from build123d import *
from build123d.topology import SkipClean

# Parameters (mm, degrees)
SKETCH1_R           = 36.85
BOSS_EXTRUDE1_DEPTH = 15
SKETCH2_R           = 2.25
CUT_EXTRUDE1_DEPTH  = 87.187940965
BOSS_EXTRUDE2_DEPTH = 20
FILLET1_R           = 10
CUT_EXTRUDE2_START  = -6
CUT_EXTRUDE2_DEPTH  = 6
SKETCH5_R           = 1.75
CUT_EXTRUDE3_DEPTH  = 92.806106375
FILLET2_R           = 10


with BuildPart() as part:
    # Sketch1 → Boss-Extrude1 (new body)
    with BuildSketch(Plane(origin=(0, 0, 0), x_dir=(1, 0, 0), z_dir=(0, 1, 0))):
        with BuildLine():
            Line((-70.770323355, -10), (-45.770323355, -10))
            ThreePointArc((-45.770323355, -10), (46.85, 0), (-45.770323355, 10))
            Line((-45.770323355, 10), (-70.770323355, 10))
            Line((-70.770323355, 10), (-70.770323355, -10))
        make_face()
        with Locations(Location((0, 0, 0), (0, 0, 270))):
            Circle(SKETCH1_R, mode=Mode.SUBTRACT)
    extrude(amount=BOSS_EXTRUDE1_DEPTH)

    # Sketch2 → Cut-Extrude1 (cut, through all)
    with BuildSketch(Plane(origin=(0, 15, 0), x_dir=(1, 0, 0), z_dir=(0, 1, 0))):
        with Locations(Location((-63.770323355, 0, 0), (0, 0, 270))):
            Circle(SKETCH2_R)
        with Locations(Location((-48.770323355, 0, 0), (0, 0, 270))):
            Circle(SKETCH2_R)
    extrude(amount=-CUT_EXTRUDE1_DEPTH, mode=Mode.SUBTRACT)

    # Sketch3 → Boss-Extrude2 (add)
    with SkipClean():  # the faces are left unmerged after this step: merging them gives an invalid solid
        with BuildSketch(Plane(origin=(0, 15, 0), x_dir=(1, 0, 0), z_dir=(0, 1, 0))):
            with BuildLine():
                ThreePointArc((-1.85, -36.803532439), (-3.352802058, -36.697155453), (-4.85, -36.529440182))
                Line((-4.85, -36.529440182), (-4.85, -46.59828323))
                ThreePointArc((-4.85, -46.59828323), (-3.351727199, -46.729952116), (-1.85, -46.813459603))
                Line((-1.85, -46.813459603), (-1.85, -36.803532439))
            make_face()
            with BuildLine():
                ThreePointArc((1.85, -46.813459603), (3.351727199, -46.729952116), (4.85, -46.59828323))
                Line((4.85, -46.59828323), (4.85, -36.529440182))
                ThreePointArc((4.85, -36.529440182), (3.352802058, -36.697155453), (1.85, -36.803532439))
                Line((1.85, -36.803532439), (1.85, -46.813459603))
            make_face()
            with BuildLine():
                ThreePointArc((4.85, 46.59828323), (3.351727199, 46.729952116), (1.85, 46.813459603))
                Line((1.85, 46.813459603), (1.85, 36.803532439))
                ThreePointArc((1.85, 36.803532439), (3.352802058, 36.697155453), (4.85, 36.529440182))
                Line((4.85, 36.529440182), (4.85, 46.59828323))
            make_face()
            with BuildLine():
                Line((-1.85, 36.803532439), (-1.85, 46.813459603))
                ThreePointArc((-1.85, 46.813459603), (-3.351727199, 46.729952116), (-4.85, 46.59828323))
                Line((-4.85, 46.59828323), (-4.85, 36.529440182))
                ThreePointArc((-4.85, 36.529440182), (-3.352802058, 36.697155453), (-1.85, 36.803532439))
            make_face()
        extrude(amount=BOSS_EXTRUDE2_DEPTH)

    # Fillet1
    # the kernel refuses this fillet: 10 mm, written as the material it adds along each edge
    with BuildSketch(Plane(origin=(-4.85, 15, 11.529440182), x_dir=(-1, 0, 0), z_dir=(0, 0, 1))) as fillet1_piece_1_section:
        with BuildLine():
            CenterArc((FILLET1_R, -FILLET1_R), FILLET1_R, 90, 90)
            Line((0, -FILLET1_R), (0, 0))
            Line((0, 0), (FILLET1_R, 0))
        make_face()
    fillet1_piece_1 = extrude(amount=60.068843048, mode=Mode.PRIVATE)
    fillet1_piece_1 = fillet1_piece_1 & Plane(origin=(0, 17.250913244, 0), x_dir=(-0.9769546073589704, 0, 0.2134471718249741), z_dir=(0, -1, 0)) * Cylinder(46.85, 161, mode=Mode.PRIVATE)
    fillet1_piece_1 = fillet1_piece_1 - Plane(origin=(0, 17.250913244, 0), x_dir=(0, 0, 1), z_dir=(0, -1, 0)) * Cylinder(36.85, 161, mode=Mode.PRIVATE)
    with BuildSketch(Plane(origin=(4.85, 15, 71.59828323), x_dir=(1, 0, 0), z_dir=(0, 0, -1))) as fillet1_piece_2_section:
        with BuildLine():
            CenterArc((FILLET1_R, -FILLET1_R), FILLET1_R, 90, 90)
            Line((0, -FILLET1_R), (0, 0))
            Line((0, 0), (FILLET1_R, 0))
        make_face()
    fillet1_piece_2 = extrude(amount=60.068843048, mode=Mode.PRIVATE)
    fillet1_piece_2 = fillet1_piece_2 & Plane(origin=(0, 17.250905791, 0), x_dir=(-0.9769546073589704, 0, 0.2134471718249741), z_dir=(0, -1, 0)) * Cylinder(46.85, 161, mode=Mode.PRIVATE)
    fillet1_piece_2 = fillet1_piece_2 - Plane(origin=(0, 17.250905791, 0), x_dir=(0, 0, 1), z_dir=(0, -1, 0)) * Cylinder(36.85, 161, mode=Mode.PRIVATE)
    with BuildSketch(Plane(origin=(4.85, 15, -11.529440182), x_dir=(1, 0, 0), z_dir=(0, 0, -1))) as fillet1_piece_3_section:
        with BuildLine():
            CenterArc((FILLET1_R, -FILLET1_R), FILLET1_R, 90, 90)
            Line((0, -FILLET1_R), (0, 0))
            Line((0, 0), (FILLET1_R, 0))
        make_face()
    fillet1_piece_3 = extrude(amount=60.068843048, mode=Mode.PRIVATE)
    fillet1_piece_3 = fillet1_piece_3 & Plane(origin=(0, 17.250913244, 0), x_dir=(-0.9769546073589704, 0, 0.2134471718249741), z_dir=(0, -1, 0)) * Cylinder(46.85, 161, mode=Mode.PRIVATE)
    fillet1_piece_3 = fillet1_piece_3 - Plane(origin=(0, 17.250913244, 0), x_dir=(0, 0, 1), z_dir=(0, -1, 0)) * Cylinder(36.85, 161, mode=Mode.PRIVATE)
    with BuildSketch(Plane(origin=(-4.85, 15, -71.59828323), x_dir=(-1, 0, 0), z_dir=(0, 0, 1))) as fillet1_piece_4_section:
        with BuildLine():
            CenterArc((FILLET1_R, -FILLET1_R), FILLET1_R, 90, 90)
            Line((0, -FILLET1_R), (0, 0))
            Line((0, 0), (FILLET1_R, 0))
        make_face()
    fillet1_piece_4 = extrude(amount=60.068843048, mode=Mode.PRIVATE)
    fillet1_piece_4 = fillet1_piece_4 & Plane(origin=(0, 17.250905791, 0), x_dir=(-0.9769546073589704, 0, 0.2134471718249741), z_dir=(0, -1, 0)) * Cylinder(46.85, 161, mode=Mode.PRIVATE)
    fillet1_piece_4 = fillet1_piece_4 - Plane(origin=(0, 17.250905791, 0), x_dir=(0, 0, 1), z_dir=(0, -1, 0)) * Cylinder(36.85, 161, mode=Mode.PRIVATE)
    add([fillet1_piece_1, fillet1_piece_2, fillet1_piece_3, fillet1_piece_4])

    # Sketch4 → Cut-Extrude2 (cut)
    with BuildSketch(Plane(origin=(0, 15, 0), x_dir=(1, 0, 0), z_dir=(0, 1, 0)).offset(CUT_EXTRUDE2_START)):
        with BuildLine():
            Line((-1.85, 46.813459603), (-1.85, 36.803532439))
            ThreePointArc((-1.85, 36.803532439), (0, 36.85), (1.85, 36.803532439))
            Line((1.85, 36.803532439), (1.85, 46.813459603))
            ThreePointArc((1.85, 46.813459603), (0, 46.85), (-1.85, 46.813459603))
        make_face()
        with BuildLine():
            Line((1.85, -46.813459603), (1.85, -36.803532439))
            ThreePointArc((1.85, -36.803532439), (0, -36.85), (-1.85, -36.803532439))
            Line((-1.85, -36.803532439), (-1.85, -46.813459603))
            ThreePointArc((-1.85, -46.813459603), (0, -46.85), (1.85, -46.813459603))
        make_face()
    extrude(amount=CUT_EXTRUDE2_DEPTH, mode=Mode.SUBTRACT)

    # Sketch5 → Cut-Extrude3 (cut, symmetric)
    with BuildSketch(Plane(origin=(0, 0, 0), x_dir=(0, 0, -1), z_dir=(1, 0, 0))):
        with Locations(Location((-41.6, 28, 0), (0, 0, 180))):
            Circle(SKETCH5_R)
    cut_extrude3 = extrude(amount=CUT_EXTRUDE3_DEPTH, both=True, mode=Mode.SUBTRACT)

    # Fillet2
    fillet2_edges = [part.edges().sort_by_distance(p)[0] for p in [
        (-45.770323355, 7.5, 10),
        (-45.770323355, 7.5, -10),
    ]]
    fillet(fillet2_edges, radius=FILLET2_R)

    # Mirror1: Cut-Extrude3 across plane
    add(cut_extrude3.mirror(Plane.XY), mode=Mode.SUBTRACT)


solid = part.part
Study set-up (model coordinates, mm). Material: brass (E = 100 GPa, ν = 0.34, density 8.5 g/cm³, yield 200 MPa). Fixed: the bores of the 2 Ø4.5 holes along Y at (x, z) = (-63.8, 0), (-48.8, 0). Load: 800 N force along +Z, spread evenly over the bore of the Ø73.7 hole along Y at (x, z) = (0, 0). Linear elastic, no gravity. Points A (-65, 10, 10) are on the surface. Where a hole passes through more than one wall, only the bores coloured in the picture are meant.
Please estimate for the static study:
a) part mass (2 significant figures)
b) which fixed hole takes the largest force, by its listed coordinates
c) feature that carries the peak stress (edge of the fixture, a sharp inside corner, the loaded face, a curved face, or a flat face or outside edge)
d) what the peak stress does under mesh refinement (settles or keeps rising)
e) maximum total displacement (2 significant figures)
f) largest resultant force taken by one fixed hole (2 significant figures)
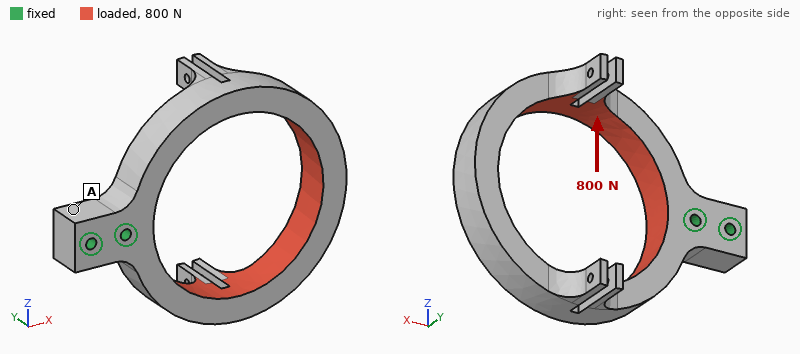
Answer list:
420 g
(-48.8, 0)
edge of the fixture
keeps rising
0.24 mm
2.5 kN
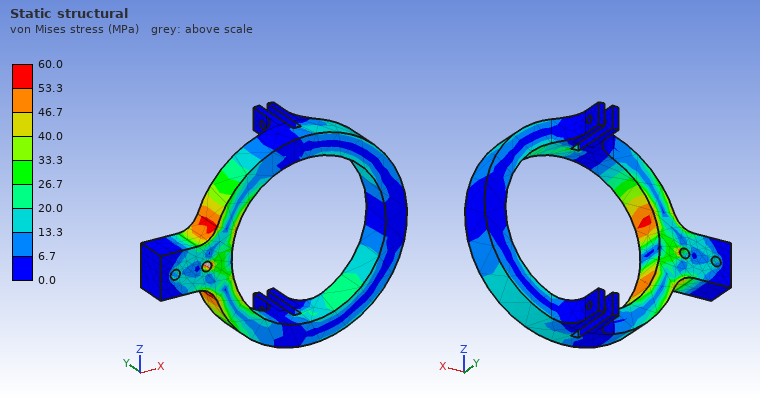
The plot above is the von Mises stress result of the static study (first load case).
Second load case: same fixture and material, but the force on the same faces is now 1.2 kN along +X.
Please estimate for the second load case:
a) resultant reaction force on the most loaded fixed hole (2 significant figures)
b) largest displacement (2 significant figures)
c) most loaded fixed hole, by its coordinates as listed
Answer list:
640 N
47 µm
(-63.8, 0)
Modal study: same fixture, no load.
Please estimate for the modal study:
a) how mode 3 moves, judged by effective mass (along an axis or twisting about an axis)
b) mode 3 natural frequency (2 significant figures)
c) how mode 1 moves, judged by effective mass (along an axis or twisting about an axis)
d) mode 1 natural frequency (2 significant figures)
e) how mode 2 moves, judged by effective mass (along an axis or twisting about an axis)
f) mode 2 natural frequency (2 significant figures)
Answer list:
twisting about X
1100 Hz
along Y
460 Hz
along Z
530 Hz
